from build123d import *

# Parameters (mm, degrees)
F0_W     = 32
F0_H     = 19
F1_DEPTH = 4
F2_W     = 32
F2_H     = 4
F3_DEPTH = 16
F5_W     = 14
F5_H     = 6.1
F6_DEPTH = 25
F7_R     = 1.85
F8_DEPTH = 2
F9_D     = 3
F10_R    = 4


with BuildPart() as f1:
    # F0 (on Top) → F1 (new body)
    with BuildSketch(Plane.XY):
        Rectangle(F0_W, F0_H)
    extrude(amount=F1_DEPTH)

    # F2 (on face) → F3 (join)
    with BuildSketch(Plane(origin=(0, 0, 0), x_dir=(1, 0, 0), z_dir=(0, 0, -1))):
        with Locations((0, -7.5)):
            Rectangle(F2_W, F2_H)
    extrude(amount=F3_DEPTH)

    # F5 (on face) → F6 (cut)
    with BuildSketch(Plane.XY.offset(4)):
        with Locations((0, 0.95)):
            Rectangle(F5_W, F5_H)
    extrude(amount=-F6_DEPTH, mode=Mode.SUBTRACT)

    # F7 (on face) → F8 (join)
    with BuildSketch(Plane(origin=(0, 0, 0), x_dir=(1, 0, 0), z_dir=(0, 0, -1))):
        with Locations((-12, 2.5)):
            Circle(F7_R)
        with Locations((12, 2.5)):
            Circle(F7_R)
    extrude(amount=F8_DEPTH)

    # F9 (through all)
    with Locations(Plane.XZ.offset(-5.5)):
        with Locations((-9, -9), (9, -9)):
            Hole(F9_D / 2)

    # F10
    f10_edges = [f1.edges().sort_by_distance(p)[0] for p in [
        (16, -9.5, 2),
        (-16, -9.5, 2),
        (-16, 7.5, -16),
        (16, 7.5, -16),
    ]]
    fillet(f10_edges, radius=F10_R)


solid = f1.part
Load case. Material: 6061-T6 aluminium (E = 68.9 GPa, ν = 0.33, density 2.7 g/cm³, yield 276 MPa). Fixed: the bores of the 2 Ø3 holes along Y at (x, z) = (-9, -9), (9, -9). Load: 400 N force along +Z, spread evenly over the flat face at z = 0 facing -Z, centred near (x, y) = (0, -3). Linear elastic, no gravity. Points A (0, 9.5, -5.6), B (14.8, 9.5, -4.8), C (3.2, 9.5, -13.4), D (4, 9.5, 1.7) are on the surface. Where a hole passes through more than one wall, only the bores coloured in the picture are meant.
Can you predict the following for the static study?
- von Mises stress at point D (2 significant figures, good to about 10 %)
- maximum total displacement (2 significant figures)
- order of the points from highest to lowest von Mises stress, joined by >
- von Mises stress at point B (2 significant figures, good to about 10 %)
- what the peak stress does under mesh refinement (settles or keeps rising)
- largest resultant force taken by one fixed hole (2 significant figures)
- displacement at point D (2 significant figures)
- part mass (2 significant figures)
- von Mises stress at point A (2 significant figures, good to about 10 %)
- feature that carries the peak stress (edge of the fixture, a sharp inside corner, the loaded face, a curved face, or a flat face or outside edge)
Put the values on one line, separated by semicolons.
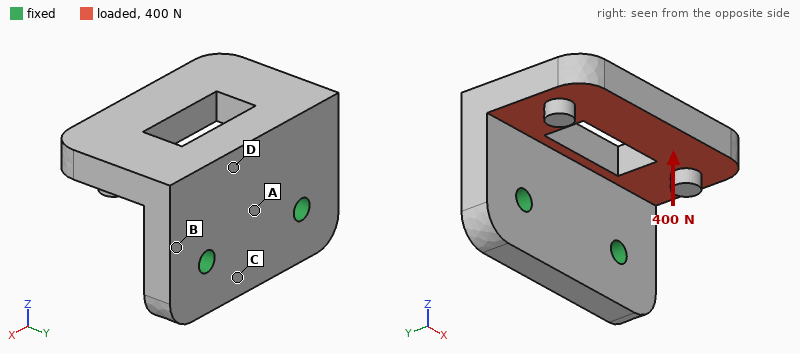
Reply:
18 MPa; 0.11 mm; B > A > D > C; 44 MPa; keeps rising; 200 N; 0.022 mm; 11 g; 30 MPa; edge of the fixture
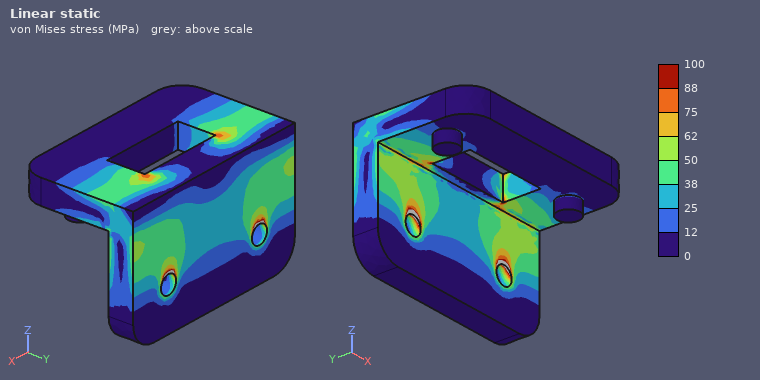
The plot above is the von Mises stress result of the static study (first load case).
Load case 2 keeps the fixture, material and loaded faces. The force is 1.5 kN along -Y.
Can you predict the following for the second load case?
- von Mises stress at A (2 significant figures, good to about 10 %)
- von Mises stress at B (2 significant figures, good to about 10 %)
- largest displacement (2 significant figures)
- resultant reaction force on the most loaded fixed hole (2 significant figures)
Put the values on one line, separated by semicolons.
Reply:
54 MPa; 69 MPa; 81 µm; 750 N
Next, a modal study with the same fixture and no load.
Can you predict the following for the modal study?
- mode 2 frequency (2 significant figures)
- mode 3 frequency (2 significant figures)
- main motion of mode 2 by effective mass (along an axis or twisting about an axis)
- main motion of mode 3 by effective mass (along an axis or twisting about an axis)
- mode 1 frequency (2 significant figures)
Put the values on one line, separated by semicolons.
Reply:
8800 Hz; 13 kHz; along X; along Y; 5200 Hz
